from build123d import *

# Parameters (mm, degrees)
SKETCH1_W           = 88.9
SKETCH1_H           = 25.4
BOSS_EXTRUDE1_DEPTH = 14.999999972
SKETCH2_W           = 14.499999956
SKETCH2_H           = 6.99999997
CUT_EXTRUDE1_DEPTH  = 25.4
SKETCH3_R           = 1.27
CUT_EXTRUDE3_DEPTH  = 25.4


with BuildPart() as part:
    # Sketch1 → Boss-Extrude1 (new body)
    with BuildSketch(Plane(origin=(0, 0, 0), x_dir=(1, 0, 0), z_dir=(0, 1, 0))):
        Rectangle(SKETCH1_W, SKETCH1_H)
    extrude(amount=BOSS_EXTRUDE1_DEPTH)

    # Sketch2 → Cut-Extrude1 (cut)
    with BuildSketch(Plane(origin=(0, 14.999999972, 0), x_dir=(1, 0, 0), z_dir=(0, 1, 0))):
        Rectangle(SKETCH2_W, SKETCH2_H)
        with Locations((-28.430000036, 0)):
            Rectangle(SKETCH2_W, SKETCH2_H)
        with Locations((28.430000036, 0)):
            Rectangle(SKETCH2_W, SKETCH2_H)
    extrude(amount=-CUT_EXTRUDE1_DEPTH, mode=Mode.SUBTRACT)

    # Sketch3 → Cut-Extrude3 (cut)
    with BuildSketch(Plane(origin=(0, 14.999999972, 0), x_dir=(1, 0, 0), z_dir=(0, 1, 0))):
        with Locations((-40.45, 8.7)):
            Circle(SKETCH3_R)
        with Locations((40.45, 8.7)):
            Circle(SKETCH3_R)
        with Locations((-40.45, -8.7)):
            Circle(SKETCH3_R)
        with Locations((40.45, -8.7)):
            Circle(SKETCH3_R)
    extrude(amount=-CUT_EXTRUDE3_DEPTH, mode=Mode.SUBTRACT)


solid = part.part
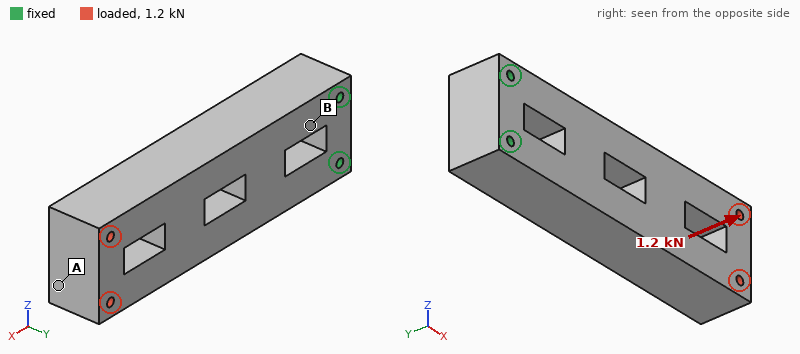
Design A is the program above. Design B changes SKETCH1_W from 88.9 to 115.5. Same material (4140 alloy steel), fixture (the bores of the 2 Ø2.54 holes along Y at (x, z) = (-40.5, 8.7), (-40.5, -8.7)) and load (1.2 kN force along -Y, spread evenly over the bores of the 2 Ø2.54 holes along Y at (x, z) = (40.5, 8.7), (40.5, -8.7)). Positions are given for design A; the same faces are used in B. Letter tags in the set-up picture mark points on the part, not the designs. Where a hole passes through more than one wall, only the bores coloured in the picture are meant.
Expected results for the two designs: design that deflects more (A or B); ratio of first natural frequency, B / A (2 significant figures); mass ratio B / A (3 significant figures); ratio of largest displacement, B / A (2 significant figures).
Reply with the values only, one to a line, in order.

B
0.73
1.35
1.2
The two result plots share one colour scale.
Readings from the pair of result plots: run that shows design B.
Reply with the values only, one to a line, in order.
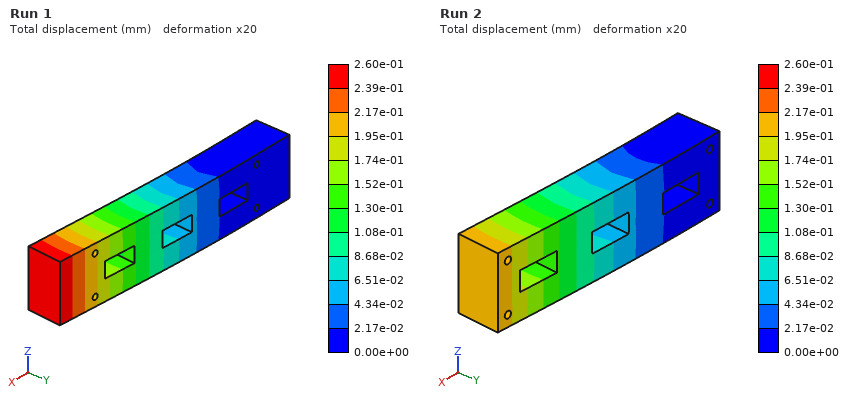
Run 1
